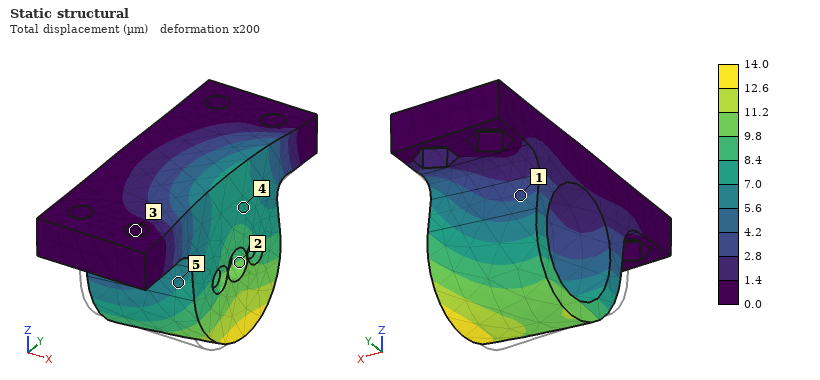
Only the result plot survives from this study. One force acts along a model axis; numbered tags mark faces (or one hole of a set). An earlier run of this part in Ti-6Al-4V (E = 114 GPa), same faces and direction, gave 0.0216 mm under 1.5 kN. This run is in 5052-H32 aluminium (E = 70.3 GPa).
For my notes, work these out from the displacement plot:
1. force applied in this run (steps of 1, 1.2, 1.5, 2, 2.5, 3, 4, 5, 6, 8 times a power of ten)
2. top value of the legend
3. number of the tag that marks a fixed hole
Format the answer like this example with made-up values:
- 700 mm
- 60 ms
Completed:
- 600 N
- 14.0 µm
- 3
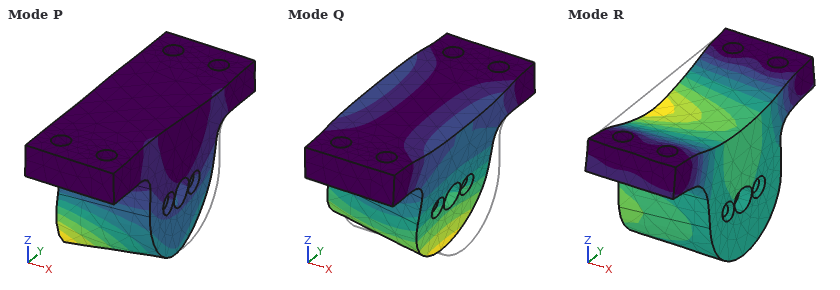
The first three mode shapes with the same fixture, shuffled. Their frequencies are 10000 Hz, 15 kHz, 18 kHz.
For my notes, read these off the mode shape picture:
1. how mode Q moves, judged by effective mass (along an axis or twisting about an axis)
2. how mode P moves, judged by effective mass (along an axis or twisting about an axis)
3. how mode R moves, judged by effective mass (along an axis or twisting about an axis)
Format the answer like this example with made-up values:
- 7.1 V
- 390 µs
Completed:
- along X
- along Y
- along Z
